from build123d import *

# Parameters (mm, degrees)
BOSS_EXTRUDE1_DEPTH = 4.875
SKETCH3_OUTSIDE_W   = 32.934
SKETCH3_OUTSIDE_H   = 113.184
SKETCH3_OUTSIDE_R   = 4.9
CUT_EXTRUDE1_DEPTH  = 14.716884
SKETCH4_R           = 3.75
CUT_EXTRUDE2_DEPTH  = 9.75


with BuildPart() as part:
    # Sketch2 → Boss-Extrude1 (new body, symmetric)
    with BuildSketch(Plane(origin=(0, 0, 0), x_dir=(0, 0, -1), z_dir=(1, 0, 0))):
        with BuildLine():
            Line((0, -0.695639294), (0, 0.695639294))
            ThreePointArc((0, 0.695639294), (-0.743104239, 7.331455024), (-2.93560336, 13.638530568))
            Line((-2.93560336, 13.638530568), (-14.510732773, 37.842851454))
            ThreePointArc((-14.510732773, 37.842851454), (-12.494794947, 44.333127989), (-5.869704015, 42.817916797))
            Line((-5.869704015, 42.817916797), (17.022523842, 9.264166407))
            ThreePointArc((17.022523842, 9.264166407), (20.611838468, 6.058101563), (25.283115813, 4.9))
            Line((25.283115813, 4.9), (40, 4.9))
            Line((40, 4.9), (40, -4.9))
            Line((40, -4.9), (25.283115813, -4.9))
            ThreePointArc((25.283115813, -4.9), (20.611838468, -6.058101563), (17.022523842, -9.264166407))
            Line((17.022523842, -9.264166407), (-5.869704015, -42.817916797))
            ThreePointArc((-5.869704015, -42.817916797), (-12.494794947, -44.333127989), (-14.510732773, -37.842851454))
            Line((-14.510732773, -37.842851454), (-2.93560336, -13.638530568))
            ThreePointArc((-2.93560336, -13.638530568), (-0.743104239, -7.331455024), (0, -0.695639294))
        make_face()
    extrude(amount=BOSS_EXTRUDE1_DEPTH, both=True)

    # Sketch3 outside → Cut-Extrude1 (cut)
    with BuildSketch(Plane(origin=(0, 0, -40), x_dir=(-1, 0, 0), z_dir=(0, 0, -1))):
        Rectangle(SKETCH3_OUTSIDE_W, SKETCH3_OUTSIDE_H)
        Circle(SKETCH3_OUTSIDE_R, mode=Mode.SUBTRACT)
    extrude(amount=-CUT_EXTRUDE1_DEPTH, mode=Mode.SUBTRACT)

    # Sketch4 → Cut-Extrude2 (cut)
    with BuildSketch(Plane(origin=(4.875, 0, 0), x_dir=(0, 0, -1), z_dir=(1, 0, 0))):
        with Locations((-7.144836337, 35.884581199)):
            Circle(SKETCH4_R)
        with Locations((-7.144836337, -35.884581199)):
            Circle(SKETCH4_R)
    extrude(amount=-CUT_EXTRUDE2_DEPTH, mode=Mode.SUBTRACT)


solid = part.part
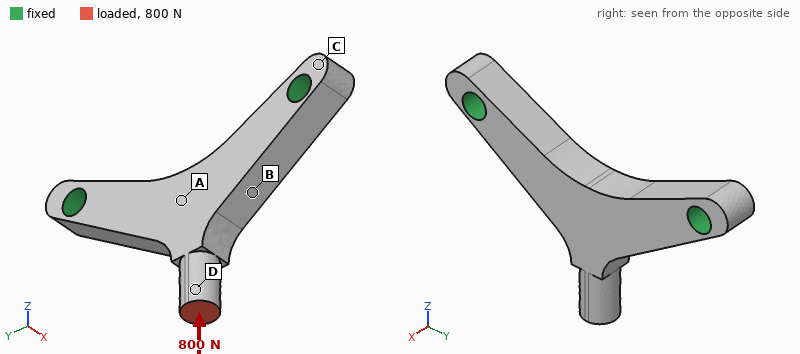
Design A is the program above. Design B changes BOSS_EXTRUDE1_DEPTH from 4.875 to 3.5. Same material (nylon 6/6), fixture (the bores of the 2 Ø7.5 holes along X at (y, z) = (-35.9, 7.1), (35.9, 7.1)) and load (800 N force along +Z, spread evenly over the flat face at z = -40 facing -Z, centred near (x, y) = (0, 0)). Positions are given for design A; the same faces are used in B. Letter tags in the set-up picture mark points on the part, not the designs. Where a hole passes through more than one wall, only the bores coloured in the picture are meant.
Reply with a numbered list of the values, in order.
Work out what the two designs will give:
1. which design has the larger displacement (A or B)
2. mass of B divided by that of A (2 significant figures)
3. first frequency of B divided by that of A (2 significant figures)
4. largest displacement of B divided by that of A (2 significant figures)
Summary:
1. B
2. 0.73
3. 0.74
4. 1.3
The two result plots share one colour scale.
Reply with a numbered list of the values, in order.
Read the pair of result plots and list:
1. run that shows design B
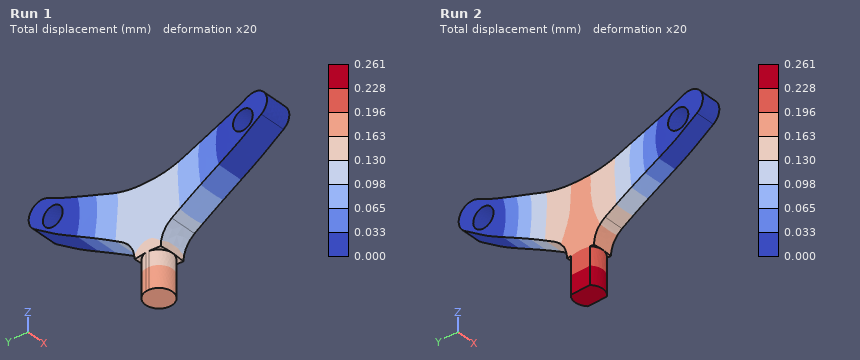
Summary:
1. Run 2
